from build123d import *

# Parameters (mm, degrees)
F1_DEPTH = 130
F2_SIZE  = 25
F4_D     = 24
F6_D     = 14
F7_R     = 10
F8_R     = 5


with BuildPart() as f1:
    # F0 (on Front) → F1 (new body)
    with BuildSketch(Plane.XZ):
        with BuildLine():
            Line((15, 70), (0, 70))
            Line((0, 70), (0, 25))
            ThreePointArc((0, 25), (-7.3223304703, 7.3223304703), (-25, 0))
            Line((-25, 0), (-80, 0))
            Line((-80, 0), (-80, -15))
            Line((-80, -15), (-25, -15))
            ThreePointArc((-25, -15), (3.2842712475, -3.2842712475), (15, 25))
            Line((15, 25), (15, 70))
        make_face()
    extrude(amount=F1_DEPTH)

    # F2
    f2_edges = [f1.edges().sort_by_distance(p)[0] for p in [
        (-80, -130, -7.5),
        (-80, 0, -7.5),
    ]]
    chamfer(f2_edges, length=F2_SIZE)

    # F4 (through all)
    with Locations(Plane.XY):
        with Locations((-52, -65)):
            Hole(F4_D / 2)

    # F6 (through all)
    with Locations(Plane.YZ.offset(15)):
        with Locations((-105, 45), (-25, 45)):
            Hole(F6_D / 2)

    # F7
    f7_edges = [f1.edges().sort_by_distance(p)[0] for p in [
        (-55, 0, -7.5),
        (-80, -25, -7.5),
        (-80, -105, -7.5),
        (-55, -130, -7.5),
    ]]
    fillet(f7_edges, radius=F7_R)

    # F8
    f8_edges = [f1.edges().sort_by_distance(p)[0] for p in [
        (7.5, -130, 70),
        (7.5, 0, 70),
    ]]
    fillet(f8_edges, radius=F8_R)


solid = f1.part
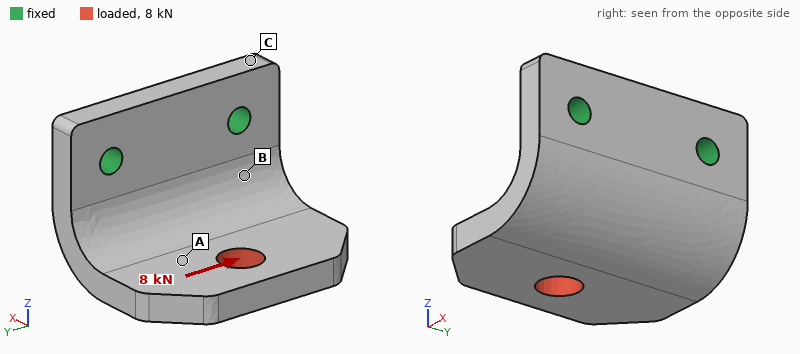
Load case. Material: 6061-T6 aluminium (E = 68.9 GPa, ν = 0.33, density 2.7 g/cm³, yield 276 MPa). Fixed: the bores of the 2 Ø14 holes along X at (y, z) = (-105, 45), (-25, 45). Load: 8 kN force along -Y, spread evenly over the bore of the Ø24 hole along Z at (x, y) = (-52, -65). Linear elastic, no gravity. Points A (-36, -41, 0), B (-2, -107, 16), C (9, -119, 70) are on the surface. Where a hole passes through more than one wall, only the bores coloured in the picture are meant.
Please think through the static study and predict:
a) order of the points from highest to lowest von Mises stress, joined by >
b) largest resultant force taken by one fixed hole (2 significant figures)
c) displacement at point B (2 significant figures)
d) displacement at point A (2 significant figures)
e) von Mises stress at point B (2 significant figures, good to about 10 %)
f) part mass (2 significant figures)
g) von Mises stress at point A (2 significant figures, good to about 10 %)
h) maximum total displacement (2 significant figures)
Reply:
B > A > C
8.0 kN
0.044 mm
0.10 mm
37 MPa
740 g
19 MPa
0.21 mm
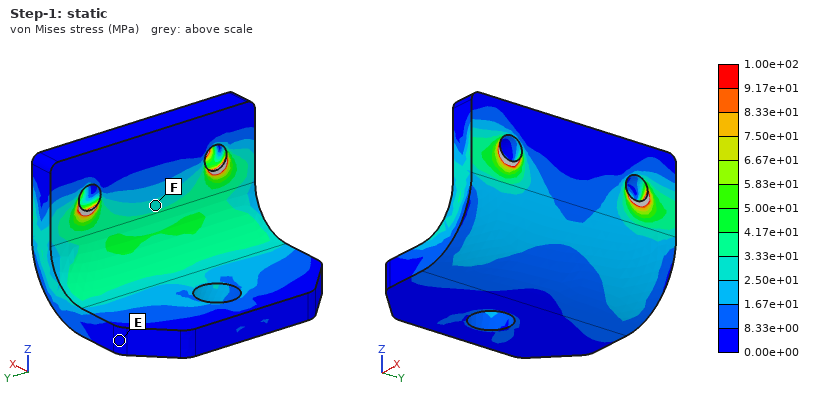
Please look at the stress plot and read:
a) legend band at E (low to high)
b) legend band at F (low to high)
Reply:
0.00e+00 to 8.33e+00 MPa
2.50e+01 to 3.33e+01 MPa
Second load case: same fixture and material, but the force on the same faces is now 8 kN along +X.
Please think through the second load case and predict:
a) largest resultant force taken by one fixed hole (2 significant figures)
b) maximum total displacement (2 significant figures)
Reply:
4.0 kN
0.44 mm
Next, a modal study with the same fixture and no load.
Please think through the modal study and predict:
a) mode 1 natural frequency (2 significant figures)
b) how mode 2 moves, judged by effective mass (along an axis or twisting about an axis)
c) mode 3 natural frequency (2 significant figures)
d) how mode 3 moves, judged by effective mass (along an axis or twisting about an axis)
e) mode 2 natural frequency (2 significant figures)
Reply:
980 Hz
along Y
3200 Hz
along X
1800 Hz
